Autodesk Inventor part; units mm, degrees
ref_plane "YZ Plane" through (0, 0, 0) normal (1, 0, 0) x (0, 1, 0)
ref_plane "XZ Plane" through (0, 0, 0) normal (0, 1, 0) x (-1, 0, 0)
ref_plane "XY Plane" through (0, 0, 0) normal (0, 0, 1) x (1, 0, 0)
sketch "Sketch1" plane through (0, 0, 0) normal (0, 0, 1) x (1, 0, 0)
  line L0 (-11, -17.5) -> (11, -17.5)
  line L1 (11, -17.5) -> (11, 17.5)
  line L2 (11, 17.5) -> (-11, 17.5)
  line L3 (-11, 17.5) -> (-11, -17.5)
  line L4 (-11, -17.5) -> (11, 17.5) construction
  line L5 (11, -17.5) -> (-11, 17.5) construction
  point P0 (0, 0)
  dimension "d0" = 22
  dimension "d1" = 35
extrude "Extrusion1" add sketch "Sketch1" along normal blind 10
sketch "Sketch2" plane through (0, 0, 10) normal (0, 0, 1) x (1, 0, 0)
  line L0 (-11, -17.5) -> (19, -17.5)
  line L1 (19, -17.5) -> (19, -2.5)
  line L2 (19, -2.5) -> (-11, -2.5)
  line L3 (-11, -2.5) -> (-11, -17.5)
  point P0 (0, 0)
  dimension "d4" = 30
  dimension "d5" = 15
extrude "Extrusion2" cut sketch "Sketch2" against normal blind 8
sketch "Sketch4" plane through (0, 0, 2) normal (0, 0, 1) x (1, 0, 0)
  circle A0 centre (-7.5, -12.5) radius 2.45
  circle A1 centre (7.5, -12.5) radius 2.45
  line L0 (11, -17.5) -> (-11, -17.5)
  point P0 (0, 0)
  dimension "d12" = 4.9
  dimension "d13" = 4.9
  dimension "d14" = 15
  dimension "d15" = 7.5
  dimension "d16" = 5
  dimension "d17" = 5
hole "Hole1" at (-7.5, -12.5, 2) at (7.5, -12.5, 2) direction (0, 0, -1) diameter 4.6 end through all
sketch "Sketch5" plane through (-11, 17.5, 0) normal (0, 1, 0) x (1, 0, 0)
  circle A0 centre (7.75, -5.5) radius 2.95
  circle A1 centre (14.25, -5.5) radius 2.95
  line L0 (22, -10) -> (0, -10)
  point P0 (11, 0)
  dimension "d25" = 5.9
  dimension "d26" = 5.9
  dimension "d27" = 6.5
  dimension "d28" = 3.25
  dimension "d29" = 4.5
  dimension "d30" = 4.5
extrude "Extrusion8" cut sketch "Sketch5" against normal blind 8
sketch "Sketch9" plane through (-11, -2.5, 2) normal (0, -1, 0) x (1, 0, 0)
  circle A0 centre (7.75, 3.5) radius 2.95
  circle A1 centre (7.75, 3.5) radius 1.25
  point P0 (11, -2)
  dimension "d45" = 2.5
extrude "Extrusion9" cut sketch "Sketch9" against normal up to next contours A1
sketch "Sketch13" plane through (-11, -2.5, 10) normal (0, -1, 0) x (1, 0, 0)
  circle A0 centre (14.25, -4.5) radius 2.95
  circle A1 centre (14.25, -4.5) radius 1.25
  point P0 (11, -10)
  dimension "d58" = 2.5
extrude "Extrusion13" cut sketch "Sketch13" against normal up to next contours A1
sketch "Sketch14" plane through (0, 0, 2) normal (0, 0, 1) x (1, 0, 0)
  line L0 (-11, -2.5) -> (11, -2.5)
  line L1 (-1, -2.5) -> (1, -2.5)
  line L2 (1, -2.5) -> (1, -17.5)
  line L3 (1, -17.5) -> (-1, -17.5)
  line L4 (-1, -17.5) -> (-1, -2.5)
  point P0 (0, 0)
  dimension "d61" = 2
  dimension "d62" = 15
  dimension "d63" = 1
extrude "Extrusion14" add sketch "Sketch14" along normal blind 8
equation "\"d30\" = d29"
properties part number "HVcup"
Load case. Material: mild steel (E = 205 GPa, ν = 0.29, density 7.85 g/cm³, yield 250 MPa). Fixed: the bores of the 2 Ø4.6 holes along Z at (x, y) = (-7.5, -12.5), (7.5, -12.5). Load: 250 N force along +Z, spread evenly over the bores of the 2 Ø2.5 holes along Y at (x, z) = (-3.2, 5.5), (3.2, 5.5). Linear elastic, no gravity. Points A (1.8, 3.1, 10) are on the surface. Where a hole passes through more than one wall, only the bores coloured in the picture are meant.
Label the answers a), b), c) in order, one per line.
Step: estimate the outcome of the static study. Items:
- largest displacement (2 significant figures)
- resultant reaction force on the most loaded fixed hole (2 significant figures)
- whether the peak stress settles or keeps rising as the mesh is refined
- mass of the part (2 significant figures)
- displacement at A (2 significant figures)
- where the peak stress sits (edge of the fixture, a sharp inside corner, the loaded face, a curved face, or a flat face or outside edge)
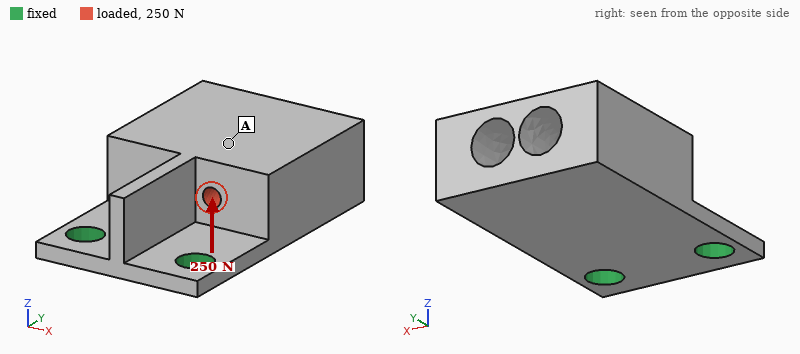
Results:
a) 62 µm
b) 130 N
c) keeps rising
d) 37 g
e) 34 µm
f) edge of the fixture
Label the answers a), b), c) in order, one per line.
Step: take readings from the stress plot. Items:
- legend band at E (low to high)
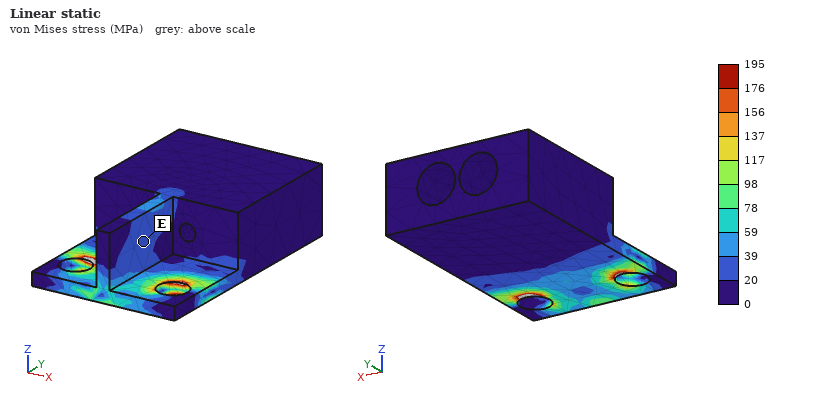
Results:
a) 20 to 39 MPa
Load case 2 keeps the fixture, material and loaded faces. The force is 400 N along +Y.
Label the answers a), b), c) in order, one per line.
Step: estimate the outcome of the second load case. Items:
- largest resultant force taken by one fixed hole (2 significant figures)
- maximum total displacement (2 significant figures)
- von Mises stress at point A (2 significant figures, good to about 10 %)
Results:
a) 200 N
b) 32 µm
c) 7.7 MPa
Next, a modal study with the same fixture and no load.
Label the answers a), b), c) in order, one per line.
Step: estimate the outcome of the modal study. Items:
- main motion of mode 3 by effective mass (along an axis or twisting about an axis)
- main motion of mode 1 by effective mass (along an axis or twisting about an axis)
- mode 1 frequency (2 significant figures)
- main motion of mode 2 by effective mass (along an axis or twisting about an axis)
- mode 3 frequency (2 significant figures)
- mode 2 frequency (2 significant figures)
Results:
a) along X
b) along Z
c) 2000 Hz
d) along X
e) 9300 Hz
f) 5100 Hz
